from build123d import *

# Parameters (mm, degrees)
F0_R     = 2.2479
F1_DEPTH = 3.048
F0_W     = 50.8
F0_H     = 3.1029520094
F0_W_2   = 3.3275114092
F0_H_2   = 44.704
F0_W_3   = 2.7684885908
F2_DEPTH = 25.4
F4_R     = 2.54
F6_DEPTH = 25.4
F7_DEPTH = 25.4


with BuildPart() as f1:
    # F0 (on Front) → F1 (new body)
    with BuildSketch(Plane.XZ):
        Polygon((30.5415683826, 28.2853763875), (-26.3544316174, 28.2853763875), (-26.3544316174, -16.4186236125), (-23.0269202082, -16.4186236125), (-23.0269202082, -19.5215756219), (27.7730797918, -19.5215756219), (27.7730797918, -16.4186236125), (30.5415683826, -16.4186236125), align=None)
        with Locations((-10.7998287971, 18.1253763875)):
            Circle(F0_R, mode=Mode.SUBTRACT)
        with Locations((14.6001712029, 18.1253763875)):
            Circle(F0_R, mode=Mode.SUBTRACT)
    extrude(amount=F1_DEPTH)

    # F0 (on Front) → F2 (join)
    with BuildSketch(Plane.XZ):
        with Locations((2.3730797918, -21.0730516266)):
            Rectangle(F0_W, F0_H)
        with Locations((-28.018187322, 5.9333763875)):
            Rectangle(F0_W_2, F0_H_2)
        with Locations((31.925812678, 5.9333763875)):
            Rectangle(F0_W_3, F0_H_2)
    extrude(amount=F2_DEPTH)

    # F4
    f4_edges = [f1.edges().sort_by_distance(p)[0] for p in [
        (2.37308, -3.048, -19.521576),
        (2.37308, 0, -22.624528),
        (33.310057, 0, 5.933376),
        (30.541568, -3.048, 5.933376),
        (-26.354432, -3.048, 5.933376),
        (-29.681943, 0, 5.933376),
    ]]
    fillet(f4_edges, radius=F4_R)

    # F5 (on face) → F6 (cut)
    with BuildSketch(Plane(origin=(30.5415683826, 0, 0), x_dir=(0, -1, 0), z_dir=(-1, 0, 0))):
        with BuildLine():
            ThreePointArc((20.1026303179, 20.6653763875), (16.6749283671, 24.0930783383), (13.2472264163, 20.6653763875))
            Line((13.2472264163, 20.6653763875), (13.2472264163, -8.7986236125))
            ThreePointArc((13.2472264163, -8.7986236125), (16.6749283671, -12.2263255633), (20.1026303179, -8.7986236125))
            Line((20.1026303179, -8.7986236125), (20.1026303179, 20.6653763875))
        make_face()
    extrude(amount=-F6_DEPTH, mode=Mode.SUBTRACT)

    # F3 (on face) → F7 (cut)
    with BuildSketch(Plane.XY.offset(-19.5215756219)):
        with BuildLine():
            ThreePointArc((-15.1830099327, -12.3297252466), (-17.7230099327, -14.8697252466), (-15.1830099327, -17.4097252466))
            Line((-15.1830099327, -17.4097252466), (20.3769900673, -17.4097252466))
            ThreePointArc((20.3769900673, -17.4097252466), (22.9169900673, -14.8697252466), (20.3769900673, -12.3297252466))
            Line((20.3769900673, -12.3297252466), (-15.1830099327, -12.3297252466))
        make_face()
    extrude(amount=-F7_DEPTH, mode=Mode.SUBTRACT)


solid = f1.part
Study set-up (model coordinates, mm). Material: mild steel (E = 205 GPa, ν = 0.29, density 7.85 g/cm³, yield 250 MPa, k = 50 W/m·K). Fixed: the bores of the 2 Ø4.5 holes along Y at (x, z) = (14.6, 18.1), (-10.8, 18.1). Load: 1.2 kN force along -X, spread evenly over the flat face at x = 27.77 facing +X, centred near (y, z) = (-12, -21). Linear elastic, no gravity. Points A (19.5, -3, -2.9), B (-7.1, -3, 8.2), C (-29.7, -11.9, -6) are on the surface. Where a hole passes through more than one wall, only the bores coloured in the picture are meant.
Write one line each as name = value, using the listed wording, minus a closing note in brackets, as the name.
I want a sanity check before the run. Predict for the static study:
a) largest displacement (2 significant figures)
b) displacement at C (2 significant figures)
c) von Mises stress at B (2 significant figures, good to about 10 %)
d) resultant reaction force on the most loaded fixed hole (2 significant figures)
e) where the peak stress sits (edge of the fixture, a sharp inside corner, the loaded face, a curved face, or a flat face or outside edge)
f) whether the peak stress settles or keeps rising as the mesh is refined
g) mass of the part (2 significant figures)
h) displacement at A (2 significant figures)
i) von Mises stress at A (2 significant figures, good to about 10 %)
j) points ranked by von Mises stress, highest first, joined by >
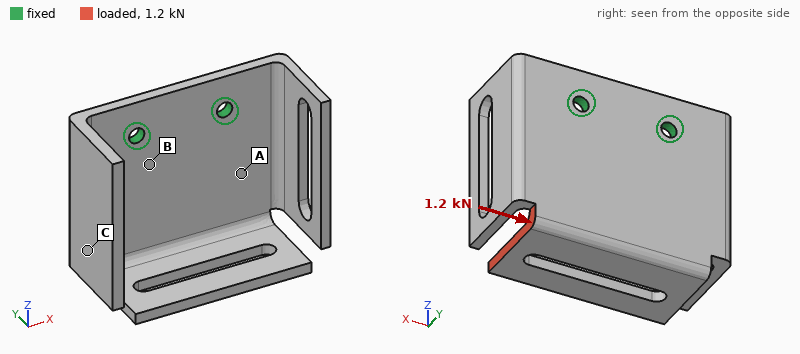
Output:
largest displacement = 0.20 mm
displacement at C = 0.11 mm
von Mises stress at B = 97 MPa
resultant reaction force on the most loaded fixed hole = 1.8 kN
where the peak stress sits = edge of the fixture
whether the peak stress settles or keeps rising as the mesh is refined = keeps rising
mass of the part = 140 g
displacement at A = 0.051 mm
von Mises stress at A = 54 MPa
points ranked by von Mises stress, highest first, joined by > = B > A > C
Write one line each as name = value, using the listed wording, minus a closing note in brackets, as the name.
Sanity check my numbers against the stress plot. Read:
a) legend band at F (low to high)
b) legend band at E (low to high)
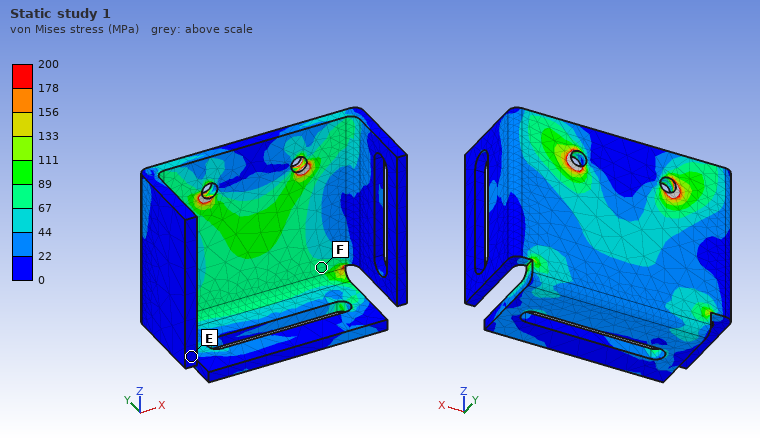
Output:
legend band at F = 67 to 89 MPa
legend band at E = 0 to 22 MPa
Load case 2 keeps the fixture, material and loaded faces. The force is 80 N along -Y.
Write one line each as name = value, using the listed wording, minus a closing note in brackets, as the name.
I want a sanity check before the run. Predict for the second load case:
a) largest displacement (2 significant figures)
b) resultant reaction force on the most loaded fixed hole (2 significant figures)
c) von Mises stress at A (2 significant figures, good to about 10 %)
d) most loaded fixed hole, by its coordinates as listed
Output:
largest displacement = 72 µm
resultant reaction force on the most loaded fixed hole = 95 N
von Mises stress at A = 5.1 MPa
most loaded fixed hole, by its coordinates as listed = (14.6, 18.1)
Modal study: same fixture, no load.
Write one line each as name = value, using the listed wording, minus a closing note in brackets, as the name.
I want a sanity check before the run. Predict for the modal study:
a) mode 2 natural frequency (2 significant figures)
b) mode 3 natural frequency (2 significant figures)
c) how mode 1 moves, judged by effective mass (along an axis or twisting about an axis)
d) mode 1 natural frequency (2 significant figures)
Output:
mode 2 natural frequency = 1300 Hz
mode 3 natural frequency = 2200 Hz
how mode 1 moves, judged by effective mass = along Y
mode 1 natural frequency = 1000 Hz
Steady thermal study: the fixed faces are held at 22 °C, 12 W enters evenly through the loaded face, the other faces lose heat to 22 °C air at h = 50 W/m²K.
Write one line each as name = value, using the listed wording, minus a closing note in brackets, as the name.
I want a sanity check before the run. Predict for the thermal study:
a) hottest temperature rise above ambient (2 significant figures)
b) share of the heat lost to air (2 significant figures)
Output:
hottest temperature rise above ambient = 82 K
share of the heat lost to air = 67 %
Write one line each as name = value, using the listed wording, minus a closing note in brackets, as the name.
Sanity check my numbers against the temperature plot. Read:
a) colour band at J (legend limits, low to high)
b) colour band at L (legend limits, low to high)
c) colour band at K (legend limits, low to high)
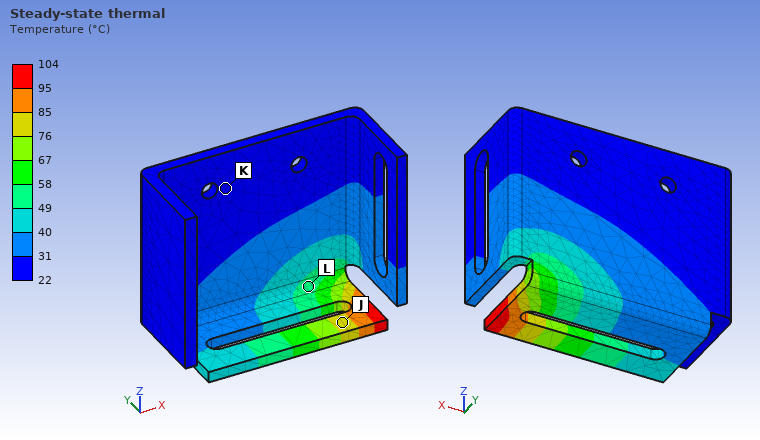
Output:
colour band at J = 76 to 85 °C
colour band at L = 49 to 58 °C
colour band at K = 22 to 31 °C
